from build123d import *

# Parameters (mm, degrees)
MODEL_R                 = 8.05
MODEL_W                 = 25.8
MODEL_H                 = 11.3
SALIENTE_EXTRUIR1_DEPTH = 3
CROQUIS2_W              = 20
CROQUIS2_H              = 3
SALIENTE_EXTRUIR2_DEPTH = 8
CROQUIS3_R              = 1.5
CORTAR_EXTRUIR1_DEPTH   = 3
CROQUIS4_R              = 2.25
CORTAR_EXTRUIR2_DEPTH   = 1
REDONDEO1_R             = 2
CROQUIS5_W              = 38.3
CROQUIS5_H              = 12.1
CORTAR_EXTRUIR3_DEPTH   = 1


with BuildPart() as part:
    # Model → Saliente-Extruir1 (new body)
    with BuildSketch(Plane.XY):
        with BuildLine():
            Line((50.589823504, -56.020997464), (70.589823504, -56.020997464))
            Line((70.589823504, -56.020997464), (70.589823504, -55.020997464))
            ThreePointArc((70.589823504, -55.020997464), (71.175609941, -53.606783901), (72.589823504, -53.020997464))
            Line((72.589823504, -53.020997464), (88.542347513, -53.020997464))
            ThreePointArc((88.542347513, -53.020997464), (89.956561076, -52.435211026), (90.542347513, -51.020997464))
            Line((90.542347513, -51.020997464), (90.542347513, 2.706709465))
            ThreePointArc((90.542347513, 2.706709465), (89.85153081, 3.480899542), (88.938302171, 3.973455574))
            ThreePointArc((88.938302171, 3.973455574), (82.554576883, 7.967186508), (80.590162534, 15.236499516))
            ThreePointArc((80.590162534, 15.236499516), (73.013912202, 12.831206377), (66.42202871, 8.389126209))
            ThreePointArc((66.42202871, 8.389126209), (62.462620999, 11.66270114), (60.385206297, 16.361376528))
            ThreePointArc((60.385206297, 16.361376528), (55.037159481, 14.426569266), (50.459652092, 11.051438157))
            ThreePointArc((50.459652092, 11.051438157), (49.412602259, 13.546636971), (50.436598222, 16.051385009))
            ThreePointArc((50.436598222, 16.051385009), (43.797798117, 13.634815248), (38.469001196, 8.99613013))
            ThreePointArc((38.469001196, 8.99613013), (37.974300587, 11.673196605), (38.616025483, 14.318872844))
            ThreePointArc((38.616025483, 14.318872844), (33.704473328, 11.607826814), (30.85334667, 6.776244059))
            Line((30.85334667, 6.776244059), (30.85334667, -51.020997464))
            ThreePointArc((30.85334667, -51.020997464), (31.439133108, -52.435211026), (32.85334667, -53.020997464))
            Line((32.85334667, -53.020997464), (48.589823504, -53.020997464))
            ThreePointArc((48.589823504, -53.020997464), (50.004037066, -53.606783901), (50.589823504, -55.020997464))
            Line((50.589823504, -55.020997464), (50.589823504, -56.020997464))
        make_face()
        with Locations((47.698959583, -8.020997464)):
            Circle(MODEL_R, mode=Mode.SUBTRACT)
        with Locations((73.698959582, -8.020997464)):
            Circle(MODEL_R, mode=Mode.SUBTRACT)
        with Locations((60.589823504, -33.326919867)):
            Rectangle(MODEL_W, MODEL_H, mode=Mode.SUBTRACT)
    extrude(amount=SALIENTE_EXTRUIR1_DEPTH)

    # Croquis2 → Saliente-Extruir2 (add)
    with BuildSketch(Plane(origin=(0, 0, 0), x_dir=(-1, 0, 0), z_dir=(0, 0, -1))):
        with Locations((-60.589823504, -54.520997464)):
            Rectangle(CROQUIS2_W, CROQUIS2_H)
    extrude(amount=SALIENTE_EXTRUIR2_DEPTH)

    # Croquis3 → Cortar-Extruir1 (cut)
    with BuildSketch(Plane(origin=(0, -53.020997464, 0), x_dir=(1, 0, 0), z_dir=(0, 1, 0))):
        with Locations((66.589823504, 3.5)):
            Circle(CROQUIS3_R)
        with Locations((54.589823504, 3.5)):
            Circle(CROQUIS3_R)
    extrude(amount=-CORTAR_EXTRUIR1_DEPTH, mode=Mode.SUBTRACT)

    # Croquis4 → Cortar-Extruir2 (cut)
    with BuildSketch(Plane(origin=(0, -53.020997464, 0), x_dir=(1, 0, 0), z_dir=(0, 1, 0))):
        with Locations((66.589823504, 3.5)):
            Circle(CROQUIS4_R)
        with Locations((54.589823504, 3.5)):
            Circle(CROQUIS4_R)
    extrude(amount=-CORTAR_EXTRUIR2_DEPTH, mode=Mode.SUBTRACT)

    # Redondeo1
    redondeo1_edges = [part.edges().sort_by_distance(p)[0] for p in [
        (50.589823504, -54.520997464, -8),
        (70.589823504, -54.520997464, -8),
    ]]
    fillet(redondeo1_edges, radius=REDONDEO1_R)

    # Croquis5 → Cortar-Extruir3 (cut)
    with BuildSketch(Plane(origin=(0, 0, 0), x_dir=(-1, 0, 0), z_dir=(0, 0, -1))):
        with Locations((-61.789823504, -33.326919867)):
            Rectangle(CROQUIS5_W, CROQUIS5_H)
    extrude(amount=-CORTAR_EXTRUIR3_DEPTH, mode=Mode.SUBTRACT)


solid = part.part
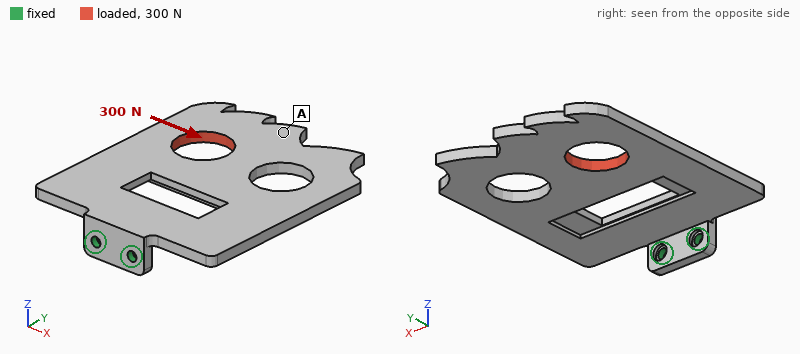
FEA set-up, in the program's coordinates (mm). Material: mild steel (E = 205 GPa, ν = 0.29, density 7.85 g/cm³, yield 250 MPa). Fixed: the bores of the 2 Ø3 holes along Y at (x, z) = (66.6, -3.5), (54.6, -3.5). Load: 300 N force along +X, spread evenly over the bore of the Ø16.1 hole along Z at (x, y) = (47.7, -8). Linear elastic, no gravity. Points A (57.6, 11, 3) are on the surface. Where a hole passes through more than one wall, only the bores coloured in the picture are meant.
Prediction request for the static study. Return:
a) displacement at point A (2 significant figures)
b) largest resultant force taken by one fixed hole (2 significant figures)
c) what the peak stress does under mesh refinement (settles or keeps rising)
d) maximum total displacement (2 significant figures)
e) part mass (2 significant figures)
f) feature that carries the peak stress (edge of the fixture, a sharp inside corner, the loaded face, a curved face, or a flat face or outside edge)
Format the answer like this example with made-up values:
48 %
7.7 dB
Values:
0.11 mm
1.1 kN
keeps rising
0.13 mm
78 g
edge of the fixture
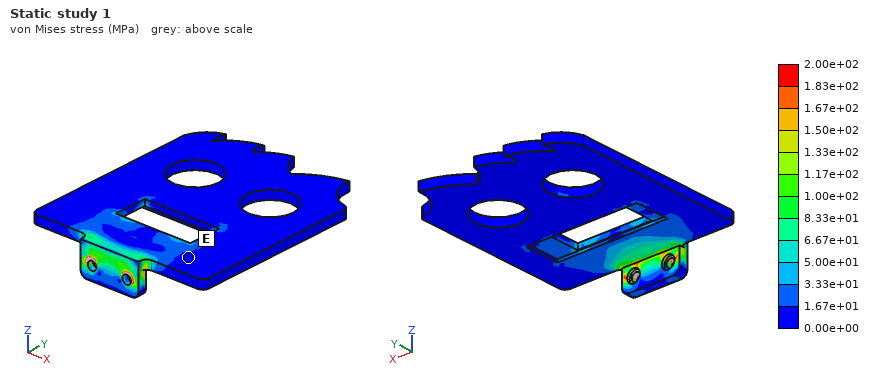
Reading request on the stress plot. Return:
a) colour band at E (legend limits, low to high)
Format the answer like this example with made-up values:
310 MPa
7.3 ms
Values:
0.00e+00 to 1.67e+01 MPa
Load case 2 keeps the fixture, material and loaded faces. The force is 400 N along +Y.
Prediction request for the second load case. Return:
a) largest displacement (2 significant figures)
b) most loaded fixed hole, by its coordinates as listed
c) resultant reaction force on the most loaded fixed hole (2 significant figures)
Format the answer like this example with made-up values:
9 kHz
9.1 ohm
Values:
73 µm
(54.6, -3.5)
580 N
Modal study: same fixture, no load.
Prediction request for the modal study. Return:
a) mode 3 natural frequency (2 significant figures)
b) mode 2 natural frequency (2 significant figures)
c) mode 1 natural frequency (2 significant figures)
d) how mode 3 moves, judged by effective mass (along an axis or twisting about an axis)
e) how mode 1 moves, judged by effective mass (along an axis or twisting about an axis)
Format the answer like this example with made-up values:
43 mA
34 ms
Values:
1300 Hz
930 Hz
330 Hz
along X
along Z
